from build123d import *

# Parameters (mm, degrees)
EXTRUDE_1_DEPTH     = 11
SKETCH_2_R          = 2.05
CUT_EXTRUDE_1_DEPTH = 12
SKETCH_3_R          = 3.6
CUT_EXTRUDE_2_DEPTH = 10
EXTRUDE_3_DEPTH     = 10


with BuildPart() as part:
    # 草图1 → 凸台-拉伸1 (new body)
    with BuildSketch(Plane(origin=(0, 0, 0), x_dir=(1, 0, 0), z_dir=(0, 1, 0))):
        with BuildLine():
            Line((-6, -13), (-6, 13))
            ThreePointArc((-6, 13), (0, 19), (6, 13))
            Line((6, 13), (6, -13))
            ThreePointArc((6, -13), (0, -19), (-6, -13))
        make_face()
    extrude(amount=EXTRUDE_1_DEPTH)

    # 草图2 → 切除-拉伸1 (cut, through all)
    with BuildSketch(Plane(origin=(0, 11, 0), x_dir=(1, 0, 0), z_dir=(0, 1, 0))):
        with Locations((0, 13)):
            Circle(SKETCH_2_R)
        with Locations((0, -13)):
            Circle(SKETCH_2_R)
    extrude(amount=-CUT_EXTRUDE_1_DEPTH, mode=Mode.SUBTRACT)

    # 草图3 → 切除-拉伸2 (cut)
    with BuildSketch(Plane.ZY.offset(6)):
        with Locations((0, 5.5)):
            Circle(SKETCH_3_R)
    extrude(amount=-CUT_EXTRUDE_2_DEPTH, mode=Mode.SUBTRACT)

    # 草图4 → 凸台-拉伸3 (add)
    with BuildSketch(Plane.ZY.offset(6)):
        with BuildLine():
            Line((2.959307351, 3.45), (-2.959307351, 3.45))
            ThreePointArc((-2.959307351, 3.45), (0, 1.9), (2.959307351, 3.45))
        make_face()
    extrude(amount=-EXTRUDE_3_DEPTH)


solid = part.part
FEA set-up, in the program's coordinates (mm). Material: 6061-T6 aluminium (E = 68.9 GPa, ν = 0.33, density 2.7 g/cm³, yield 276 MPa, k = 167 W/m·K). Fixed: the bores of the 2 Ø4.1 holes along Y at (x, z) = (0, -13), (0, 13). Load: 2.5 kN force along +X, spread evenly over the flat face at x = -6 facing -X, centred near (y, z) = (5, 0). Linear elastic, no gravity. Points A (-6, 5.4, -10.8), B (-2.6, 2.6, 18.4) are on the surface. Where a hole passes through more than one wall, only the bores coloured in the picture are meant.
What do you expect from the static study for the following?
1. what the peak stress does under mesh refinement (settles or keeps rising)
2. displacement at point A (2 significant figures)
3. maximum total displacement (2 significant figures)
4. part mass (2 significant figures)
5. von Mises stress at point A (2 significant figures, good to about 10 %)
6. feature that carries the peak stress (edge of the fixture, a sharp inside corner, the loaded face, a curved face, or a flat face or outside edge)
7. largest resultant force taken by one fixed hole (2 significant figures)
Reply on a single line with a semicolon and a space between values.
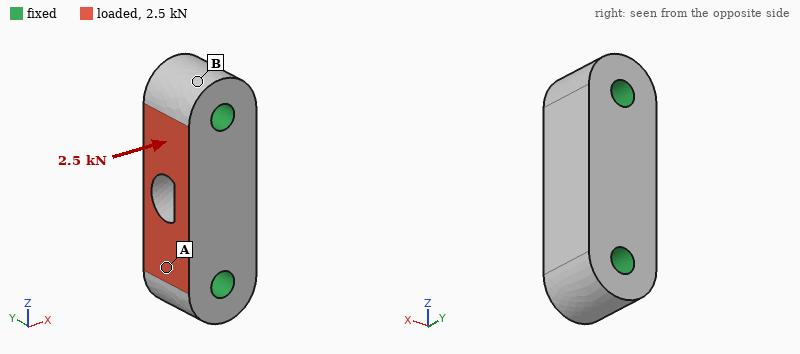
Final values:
keeps rising; 2.2 µm; 5.2 µm; 11 g; 13 MPa; edge of the fixture; 1.3 kN
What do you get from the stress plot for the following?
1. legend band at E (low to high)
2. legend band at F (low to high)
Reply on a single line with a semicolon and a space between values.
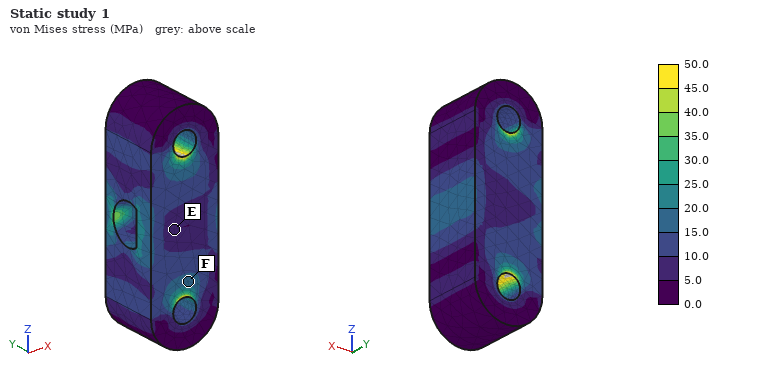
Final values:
5.0 to 10.0 MPa; 15.0 to 20.0 MPa
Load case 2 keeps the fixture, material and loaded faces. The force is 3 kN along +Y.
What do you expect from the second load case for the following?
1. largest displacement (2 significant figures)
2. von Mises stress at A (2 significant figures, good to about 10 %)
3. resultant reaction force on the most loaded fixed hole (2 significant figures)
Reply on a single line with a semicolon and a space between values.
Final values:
14 µm; 43 MPa; 1.5 kN
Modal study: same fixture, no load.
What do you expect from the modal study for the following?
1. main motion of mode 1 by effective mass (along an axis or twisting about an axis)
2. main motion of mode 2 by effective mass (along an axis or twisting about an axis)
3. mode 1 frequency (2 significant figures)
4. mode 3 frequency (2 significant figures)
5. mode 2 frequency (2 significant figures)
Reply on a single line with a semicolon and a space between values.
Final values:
along X; along Y; 47 kHz; 59 kHz; 53 kHz
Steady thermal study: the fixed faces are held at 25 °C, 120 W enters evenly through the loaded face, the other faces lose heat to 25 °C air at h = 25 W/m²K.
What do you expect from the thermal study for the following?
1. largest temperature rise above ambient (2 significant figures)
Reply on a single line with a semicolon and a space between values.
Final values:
27 K
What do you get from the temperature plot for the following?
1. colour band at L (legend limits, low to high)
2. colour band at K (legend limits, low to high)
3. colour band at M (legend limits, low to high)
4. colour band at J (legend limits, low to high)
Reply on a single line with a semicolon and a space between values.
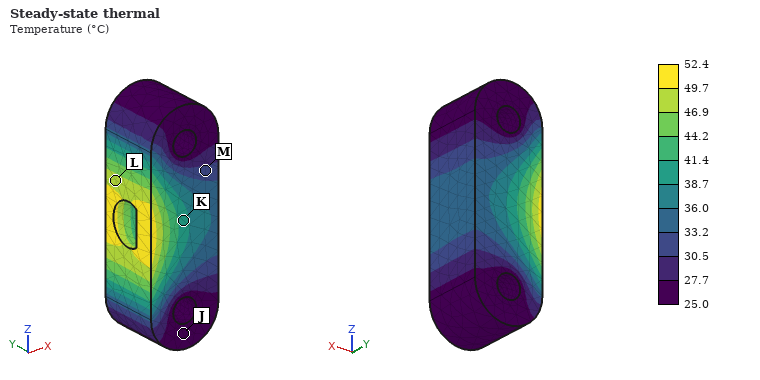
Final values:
46.9 to 49.7 °C; 38.7 to 41.4 °C; 30.5 to 33.2 °C; 25.0 to 27.7 °C
